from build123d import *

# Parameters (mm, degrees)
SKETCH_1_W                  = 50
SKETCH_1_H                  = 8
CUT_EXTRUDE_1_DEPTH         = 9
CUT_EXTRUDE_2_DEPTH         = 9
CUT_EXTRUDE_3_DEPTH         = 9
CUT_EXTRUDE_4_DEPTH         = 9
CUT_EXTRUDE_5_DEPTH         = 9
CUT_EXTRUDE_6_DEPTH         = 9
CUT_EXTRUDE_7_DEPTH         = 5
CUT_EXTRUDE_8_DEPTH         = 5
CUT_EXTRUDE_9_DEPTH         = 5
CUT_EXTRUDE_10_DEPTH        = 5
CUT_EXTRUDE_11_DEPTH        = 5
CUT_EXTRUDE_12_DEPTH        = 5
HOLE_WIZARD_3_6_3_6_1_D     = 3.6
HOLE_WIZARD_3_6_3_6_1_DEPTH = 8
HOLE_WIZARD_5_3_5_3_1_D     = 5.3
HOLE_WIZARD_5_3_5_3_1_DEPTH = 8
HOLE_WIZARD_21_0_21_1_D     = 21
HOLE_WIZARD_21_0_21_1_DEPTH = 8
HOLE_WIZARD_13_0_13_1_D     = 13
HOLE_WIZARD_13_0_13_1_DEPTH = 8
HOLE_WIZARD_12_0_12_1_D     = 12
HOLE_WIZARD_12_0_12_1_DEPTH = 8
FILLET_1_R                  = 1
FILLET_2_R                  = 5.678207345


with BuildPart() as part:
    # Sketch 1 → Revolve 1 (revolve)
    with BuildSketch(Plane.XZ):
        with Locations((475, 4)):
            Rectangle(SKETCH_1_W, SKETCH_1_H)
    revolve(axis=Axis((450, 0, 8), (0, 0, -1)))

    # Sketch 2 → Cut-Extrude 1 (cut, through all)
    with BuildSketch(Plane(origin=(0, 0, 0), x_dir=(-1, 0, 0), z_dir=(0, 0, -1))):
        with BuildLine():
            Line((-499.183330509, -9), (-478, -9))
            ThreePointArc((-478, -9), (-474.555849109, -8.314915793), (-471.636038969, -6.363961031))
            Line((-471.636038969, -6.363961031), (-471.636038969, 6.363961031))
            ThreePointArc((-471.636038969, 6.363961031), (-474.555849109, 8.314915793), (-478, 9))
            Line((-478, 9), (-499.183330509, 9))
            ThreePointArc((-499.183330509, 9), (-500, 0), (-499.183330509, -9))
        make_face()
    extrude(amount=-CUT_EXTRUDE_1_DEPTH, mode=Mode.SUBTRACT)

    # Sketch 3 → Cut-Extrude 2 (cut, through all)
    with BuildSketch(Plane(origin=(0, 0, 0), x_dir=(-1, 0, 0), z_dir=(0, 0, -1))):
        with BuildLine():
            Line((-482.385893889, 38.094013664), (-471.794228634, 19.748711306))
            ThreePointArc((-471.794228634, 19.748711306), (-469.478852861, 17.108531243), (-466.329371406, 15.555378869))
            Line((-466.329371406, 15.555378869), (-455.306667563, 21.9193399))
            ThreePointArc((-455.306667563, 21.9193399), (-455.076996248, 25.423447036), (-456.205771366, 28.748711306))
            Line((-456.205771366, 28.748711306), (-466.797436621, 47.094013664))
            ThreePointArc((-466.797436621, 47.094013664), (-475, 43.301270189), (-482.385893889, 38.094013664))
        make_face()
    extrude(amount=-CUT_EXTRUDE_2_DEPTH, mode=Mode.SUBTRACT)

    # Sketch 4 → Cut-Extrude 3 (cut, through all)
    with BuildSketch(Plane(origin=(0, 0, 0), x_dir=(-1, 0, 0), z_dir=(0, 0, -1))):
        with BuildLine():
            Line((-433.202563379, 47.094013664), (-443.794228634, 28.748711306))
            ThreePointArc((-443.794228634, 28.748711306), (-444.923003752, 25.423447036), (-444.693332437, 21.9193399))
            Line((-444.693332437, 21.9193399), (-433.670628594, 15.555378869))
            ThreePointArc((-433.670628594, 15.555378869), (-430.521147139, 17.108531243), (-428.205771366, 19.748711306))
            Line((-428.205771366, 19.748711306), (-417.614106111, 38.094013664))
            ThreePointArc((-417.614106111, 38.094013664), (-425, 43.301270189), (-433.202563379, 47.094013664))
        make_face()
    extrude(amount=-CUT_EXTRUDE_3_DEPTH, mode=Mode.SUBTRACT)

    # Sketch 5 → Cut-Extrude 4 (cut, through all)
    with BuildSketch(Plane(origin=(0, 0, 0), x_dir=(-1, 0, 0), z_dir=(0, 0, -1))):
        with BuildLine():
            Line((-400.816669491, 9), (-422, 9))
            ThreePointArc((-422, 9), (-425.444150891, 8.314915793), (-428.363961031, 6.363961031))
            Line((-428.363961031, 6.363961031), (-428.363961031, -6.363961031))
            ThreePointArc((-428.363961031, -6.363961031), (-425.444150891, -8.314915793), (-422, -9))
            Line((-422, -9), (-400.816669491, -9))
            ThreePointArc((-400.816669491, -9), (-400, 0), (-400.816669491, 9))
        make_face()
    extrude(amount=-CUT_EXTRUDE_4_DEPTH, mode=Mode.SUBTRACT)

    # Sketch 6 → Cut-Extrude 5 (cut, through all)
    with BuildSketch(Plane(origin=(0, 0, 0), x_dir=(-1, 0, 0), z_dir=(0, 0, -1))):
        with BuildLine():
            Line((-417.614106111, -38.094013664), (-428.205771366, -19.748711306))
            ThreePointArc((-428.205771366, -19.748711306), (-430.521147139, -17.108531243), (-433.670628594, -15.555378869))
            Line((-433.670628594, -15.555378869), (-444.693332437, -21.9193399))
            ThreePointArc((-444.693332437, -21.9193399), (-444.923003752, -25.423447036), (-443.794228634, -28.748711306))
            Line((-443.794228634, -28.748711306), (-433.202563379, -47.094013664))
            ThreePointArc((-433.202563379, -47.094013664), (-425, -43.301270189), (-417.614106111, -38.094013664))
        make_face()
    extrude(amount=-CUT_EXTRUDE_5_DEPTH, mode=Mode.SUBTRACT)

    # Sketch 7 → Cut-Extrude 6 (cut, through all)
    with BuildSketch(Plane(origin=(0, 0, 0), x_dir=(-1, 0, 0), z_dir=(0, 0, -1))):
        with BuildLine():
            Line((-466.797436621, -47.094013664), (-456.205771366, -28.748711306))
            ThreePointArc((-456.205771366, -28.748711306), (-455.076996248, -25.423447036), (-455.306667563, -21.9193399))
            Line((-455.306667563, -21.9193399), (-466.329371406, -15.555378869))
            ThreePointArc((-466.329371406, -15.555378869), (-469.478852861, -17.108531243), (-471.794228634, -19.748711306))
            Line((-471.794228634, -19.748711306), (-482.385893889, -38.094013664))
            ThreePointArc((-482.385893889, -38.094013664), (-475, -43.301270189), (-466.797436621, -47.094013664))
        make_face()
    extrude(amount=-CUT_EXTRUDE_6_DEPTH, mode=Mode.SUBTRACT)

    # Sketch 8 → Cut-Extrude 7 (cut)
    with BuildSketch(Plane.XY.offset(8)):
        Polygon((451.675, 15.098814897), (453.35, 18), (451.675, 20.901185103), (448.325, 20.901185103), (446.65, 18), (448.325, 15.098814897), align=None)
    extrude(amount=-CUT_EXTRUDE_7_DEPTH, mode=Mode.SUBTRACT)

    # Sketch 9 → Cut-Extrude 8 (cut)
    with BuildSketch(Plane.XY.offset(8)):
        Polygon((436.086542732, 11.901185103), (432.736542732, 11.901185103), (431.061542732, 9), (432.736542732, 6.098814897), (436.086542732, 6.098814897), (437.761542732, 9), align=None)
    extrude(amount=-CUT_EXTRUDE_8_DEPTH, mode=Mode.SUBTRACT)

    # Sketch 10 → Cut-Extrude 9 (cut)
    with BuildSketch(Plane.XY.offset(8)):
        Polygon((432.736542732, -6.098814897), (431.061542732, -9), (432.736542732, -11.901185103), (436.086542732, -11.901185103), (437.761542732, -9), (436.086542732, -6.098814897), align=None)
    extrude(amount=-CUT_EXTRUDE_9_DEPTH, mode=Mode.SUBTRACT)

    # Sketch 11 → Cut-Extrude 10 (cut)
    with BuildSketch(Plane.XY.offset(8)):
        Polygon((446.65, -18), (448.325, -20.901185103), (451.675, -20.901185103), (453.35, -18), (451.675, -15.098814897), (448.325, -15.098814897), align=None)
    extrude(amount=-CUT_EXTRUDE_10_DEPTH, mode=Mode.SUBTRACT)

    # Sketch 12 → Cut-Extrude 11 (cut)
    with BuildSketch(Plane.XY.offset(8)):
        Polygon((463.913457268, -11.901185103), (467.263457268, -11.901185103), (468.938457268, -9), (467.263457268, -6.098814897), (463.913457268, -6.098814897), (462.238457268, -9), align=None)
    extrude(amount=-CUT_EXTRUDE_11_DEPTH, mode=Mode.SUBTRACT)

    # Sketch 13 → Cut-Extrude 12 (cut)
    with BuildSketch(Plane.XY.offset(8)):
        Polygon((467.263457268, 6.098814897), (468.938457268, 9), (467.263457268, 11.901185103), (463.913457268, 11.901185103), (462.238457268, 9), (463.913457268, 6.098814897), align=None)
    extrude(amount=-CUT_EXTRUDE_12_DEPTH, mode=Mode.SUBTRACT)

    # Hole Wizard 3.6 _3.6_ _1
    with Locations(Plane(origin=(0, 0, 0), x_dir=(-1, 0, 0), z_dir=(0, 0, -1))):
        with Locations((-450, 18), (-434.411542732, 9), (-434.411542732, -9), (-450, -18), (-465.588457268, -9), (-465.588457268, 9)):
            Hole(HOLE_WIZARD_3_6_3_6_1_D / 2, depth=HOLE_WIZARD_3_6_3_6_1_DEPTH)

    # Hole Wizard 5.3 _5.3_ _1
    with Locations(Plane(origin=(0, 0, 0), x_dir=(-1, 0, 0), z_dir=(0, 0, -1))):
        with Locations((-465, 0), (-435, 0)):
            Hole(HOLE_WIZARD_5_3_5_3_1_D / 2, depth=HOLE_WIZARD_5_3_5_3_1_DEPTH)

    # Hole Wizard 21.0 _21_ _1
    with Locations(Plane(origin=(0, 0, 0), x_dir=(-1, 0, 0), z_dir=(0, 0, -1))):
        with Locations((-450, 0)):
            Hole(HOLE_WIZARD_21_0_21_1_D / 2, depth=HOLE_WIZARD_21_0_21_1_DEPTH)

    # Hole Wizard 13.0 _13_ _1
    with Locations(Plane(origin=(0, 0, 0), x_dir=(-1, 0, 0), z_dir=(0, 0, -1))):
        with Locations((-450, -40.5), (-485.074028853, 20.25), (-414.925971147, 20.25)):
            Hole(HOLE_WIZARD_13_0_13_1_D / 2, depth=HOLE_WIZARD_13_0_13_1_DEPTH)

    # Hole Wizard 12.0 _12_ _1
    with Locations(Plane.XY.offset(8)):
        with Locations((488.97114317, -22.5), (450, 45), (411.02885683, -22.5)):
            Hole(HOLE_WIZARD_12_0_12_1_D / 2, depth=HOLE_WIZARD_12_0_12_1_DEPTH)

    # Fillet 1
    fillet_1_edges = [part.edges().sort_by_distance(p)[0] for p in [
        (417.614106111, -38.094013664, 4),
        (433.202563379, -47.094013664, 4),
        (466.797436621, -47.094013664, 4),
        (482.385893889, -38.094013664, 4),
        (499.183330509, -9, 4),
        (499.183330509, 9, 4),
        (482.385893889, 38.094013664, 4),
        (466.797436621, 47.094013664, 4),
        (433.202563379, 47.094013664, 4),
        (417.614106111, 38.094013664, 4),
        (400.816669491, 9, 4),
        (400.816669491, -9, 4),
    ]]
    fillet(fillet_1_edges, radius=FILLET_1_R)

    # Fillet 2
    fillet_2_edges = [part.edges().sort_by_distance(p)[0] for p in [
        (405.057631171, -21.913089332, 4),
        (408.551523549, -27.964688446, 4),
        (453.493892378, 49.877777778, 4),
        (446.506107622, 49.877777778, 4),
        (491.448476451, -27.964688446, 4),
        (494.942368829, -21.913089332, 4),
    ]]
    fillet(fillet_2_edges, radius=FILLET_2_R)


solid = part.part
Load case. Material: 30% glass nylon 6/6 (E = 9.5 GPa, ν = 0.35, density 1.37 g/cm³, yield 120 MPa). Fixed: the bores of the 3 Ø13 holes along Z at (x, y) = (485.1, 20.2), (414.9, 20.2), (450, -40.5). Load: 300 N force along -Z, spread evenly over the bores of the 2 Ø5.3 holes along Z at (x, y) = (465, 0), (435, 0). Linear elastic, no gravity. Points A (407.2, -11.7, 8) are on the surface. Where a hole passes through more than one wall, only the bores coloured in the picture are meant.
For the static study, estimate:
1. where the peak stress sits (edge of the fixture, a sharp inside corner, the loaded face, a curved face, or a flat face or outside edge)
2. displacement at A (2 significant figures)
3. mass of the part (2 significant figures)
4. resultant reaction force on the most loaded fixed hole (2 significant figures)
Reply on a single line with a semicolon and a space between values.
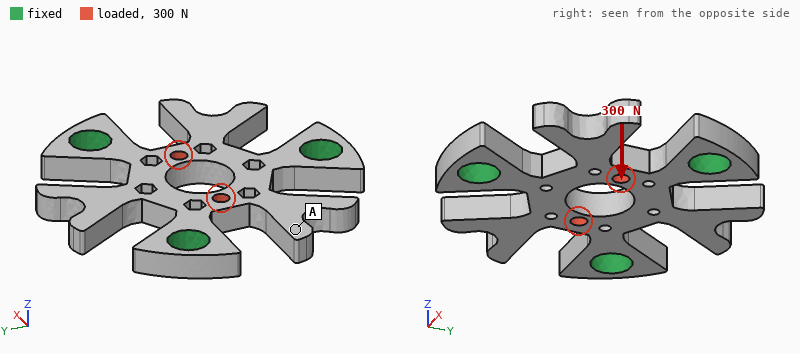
the loaded face; 59 µm; 39 g; 110 N
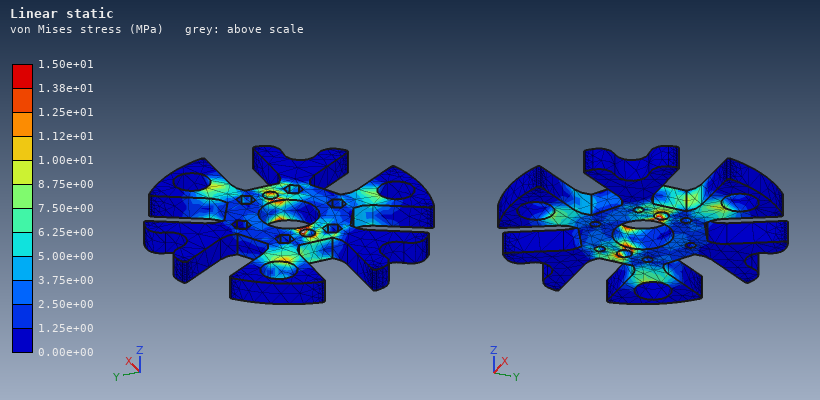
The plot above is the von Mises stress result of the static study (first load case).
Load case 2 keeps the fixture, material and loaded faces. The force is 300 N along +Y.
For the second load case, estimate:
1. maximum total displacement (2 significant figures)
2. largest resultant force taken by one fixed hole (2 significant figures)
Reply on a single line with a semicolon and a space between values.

17 µm; 110 N
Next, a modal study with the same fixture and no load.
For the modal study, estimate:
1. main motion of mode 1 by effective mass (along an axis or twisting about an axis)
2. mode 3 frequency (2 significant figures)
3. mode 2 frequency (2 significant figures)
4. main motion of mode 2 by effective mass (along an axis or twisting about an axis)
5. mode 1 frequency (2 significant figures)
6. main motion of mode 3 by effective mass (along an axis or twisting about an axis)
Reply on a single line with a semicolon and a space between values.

twisting about Y; 1500 Hz; 1300 Hz; twisting about X; 1200 Hz; along Z
